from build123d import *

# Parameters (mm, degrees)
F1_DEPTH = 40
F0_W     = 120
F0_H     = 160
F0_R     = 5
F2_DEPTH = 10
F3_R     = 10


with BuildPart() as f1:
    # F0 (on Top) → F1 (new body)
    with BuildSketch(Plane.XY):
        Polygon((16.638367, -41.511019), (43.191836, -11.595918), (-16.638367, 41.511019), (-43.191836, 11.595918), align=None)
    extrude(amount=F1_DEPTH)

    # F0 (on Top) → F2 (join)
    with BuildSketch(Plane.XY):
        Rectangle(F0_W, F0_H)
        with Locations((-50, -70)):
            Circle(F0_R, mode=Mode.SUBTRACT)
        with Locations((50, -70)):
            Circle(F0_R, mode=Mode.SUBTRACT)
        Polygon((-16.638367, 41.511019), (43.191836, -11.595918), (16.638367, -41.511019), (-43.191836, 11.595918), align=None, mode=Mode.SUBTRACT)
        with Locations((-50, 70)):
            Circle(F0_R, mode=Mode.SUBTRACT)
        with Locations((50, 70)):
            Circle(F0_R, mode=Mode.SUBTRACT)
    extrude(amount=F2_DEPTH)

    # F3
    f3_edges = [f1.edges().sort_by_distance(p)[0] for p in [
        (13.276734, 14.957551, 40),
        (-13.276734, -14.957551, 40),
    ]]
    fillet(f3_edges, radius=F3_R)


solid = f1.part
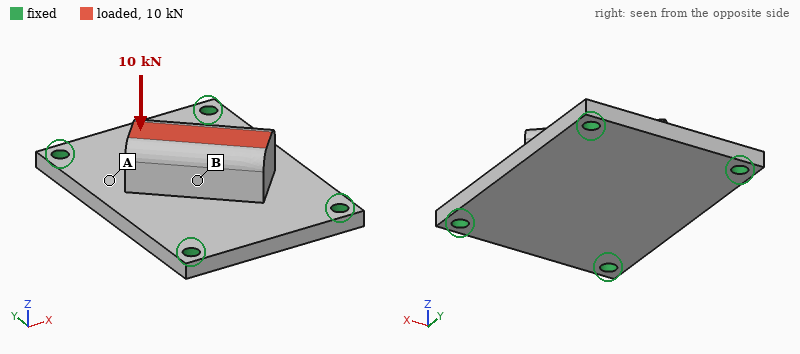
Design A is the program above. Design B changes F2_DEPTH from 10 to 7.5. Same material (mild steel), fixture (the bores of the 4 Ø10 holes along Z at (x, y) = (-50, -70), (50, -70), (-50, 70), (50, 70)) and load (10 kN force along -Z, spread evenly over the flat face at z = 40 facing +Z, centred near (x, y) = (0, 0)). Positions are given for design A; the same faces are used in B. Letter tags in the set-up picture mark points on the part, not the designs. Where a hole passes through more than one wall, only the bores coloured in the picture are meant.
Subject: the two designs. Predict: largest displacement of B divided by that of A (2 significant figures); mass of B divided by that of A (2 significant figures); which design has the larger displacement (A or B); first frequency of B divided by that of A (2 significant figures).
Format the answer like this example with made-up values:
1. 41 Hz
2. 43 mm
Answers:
1. 2.0
2. 0.86
3. B
4. 0.73
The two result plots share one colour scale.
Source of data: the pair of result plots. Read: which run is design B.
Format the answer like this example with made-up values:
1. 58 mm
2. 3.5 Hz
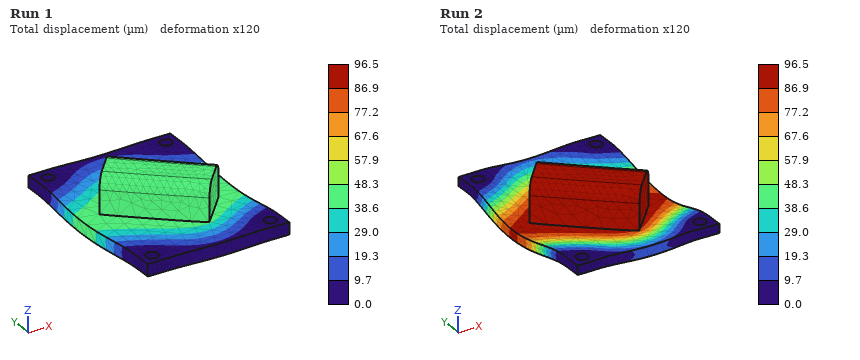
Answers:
1. Run 2
